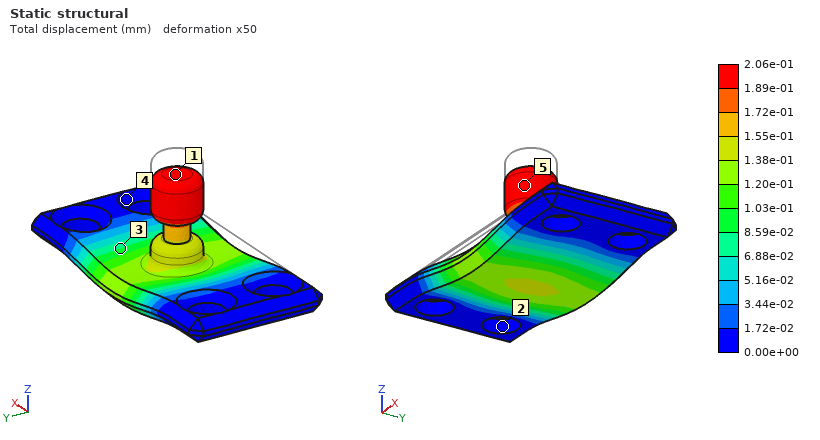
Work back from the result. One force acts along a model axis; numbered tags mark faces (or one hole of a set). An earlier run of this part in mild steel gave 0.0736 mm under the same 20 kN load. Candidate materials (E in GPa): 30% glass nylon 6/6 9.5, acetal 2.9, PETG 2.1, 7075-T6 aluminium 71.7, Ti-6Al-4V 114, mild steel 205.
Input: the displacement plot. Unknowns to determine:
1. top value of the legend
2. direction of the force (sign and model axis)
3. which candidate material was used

2.06e-01 mm
-Z
7075-T6 aluminium
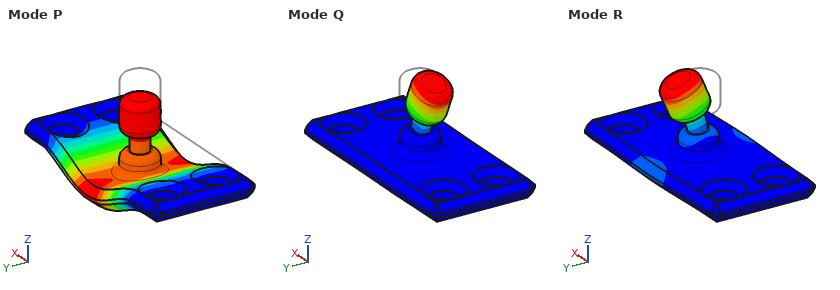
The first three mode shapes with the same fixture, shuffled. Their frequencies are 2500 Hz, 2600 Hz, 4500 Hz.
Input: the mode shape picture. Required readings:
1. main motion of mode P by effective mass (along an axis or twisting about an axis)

along Z
